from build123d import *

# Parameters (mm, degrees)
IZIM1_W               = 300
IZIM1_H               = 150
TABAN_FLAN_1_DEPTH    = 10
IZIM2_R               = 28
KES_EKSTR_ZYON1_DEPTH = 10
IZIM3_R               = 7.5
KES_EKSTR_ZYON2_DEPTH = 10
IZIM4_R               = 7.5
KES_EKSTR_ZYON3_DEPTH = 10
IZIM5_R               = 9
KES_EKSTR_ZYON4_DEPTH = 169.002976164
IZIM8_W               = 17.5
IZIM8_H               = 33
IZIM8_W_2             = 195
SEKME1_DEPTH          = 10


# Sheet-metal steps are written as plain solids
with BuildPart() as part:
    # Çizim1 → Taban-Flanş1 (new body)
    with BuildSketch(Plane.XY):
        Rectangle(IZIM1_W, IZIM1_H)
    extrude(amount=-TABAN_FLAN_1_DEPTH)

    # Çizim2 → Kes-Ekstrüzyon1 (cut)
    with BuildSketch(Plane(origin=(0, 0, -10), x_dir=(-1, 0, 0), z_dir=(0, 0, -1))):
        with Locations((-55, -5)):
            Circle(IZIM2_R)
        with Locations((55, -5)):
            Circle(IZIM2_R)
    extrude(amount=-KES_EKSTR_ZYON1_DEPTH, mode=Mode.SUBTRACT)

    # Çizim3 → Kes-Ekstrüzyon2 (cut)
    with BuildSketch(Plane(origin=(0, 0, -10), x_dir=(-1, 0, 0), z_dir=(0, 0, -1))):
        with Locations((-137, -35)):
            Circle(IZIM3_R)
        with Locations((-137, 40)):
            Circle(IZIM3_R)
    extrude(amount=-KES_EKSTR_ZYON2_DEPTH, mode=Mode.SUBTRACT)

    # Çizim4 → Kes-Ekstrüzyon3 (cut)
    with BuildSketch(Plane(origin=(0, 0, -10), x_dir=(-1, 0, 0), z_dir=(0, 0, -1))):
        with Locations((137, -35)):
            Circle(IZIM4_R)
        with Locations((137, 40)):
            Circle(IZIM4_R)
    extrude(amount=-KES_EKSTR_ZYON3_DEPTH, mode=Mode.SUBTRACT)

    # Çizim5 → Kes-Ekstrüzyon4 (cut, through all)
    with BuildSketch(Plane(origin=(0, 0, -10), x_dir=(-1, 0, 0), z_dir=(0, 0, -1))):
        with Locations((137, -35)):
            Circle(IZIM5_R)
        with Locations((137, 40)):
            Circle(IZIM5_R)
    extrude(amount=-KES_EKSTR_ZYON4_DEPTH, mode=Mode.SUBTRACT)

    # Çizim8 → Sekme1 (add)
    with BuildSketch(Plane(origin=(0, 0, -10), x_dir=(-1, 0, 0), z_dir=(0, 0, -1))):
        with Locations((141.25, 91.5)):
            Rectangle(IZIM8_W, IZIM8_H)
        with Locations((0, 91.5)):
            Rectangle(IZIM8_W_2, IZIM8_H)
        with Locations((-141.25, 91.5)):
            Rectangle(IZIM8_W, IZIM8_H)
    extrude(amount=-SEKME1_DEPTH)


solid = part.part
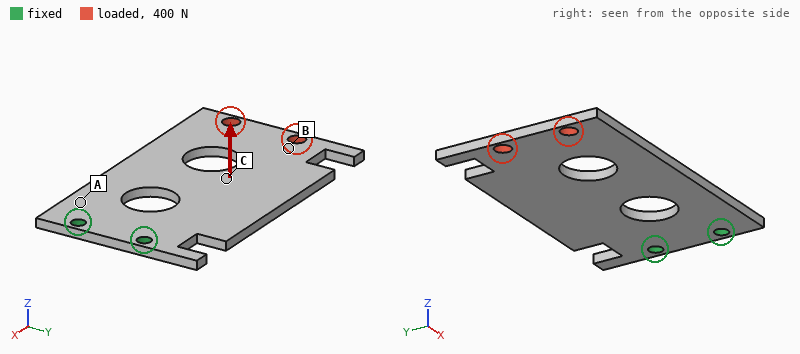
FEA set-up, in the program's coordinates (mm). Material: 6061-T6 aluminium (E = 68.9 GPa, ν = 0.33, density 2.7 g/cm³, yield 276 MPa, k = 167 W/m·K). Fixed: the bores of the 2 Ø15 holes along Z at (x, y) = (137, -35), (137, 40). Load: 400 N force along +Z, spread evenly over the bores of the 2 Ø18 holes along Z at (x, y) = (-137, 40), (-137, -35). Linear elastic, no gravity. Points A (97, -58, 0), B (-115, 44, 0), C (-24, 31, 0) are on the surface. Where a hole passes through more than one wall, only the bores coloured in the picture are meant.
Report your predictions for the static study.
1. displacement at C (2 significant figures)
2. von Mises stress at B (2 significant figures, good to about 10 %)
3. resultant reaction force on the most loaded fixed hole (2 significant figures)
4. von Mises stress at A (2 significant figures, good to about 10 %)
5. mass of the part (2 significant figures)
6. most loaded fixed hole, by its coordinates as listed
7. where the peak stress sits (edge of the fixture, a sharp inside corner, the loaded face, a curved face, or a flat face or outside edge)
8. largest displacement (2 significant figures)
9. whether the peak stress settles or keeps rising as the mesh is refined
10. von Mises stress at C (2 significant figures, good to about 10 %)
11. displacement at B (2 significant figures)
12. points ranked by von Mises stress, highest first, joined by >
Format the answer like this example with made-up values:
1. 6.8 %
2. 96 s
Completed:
1. 1.4 mm
2. 7.0 MPa
3. 220 N
4. 37 MPa
5. 1.3 kg
6. (137, 40)
7. edge of the fixture
8. 3.7 mm
9. keeps rising
10. 16 MPa
11. 3.0 mm
12. A > C > B
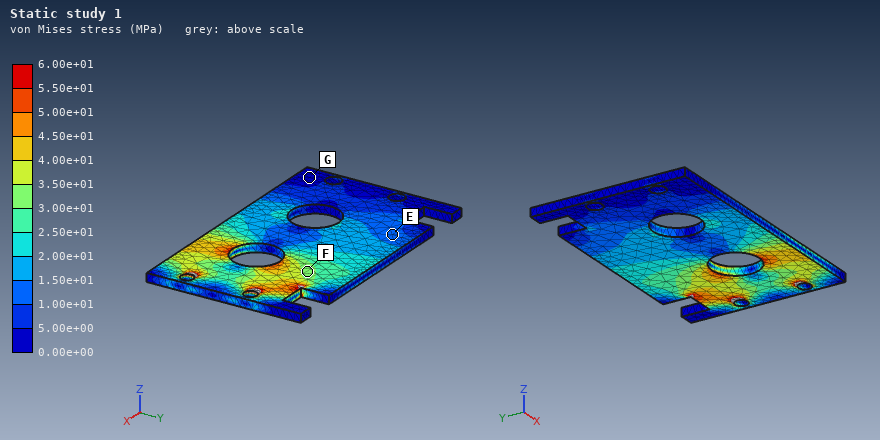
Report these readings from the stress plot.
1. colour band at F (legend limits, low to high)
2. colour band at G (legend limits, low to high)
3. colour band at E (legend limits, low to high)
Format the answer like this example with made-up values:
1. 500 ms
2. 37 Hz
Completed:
1. 3.00e+01 to 3.50e+01 MPa
2. 0.00e+00 to 5.00e+00 MPa
3. 1.00e+01 to 1.50e+01 MPa
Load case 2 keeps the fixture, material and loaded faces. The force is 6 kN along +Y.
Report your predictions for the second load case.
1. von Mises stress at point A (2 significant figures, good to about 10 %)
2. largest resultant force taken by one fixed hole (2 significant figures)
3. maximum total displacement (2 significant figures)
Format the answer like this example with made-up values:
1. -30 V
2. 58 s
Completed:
1. 31 MPa
2. 19 kN
3. 0.45 mm
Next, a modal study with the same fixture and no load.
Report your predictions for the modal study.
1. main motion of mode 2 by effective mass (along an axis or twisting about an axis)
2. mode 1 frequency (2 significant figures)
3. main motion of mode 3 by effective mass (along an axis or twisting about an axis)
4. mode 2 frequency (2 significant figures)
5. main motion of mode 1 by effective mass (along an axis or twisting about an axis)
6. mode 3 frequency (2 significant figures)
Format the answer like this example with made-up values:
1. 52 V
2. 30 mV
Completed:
1. twisting about X
2. 95 Hz
3. along Z
4. 310 Hz
5. along Z
6. 590 Hz
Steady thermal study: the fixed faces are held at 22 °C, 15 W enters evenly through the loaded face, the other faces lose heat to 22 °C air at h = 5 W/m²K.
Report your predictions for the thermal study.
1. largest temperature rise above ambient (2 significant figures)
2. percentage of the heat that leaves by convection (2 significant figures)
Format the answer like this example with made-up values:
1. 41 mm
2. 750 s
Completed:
1. 17 K
2. 26 %
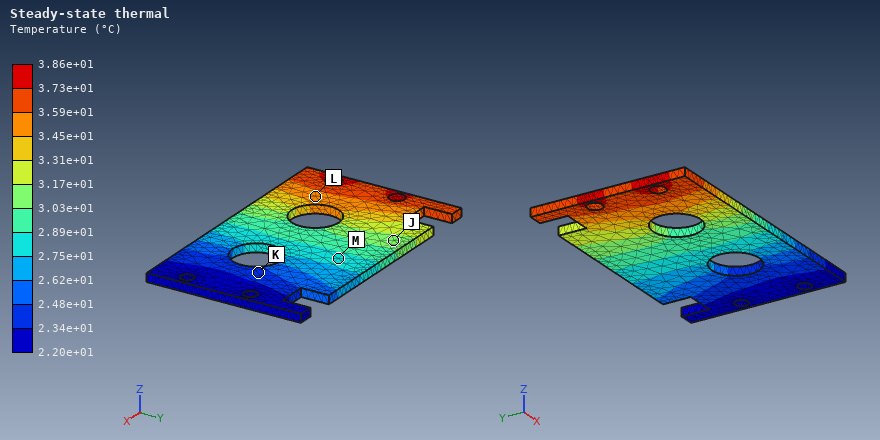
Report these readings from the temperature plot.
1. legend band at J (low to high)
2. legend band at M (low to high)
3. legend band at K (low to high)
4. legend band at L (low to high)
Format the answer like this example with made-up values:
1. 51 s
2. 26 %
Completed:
1. 3.03e+01 to 3.17e+01 °C
2. 2.75e+01 to 2.89e+01 °C
3. 2.34e+01 to 2.48e+01 °C
4. 3.45e+01 to 3.59e+01 °C
